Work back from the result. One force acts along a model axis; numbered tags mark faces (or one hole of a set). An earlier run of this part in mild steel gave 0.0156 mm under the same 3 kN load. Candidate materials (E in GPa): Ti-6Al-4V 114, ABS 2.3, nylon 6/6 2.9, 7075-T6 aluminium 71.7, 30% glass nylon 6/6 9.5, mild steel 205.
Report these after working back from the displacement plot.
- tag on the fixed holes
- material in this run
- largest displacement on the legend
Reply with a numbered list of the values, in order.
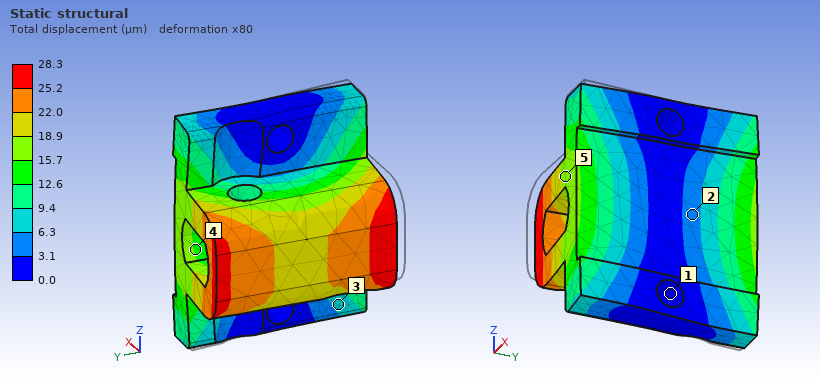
1. 1
2. Ti-6Al-4V
3. 28.3 µm
